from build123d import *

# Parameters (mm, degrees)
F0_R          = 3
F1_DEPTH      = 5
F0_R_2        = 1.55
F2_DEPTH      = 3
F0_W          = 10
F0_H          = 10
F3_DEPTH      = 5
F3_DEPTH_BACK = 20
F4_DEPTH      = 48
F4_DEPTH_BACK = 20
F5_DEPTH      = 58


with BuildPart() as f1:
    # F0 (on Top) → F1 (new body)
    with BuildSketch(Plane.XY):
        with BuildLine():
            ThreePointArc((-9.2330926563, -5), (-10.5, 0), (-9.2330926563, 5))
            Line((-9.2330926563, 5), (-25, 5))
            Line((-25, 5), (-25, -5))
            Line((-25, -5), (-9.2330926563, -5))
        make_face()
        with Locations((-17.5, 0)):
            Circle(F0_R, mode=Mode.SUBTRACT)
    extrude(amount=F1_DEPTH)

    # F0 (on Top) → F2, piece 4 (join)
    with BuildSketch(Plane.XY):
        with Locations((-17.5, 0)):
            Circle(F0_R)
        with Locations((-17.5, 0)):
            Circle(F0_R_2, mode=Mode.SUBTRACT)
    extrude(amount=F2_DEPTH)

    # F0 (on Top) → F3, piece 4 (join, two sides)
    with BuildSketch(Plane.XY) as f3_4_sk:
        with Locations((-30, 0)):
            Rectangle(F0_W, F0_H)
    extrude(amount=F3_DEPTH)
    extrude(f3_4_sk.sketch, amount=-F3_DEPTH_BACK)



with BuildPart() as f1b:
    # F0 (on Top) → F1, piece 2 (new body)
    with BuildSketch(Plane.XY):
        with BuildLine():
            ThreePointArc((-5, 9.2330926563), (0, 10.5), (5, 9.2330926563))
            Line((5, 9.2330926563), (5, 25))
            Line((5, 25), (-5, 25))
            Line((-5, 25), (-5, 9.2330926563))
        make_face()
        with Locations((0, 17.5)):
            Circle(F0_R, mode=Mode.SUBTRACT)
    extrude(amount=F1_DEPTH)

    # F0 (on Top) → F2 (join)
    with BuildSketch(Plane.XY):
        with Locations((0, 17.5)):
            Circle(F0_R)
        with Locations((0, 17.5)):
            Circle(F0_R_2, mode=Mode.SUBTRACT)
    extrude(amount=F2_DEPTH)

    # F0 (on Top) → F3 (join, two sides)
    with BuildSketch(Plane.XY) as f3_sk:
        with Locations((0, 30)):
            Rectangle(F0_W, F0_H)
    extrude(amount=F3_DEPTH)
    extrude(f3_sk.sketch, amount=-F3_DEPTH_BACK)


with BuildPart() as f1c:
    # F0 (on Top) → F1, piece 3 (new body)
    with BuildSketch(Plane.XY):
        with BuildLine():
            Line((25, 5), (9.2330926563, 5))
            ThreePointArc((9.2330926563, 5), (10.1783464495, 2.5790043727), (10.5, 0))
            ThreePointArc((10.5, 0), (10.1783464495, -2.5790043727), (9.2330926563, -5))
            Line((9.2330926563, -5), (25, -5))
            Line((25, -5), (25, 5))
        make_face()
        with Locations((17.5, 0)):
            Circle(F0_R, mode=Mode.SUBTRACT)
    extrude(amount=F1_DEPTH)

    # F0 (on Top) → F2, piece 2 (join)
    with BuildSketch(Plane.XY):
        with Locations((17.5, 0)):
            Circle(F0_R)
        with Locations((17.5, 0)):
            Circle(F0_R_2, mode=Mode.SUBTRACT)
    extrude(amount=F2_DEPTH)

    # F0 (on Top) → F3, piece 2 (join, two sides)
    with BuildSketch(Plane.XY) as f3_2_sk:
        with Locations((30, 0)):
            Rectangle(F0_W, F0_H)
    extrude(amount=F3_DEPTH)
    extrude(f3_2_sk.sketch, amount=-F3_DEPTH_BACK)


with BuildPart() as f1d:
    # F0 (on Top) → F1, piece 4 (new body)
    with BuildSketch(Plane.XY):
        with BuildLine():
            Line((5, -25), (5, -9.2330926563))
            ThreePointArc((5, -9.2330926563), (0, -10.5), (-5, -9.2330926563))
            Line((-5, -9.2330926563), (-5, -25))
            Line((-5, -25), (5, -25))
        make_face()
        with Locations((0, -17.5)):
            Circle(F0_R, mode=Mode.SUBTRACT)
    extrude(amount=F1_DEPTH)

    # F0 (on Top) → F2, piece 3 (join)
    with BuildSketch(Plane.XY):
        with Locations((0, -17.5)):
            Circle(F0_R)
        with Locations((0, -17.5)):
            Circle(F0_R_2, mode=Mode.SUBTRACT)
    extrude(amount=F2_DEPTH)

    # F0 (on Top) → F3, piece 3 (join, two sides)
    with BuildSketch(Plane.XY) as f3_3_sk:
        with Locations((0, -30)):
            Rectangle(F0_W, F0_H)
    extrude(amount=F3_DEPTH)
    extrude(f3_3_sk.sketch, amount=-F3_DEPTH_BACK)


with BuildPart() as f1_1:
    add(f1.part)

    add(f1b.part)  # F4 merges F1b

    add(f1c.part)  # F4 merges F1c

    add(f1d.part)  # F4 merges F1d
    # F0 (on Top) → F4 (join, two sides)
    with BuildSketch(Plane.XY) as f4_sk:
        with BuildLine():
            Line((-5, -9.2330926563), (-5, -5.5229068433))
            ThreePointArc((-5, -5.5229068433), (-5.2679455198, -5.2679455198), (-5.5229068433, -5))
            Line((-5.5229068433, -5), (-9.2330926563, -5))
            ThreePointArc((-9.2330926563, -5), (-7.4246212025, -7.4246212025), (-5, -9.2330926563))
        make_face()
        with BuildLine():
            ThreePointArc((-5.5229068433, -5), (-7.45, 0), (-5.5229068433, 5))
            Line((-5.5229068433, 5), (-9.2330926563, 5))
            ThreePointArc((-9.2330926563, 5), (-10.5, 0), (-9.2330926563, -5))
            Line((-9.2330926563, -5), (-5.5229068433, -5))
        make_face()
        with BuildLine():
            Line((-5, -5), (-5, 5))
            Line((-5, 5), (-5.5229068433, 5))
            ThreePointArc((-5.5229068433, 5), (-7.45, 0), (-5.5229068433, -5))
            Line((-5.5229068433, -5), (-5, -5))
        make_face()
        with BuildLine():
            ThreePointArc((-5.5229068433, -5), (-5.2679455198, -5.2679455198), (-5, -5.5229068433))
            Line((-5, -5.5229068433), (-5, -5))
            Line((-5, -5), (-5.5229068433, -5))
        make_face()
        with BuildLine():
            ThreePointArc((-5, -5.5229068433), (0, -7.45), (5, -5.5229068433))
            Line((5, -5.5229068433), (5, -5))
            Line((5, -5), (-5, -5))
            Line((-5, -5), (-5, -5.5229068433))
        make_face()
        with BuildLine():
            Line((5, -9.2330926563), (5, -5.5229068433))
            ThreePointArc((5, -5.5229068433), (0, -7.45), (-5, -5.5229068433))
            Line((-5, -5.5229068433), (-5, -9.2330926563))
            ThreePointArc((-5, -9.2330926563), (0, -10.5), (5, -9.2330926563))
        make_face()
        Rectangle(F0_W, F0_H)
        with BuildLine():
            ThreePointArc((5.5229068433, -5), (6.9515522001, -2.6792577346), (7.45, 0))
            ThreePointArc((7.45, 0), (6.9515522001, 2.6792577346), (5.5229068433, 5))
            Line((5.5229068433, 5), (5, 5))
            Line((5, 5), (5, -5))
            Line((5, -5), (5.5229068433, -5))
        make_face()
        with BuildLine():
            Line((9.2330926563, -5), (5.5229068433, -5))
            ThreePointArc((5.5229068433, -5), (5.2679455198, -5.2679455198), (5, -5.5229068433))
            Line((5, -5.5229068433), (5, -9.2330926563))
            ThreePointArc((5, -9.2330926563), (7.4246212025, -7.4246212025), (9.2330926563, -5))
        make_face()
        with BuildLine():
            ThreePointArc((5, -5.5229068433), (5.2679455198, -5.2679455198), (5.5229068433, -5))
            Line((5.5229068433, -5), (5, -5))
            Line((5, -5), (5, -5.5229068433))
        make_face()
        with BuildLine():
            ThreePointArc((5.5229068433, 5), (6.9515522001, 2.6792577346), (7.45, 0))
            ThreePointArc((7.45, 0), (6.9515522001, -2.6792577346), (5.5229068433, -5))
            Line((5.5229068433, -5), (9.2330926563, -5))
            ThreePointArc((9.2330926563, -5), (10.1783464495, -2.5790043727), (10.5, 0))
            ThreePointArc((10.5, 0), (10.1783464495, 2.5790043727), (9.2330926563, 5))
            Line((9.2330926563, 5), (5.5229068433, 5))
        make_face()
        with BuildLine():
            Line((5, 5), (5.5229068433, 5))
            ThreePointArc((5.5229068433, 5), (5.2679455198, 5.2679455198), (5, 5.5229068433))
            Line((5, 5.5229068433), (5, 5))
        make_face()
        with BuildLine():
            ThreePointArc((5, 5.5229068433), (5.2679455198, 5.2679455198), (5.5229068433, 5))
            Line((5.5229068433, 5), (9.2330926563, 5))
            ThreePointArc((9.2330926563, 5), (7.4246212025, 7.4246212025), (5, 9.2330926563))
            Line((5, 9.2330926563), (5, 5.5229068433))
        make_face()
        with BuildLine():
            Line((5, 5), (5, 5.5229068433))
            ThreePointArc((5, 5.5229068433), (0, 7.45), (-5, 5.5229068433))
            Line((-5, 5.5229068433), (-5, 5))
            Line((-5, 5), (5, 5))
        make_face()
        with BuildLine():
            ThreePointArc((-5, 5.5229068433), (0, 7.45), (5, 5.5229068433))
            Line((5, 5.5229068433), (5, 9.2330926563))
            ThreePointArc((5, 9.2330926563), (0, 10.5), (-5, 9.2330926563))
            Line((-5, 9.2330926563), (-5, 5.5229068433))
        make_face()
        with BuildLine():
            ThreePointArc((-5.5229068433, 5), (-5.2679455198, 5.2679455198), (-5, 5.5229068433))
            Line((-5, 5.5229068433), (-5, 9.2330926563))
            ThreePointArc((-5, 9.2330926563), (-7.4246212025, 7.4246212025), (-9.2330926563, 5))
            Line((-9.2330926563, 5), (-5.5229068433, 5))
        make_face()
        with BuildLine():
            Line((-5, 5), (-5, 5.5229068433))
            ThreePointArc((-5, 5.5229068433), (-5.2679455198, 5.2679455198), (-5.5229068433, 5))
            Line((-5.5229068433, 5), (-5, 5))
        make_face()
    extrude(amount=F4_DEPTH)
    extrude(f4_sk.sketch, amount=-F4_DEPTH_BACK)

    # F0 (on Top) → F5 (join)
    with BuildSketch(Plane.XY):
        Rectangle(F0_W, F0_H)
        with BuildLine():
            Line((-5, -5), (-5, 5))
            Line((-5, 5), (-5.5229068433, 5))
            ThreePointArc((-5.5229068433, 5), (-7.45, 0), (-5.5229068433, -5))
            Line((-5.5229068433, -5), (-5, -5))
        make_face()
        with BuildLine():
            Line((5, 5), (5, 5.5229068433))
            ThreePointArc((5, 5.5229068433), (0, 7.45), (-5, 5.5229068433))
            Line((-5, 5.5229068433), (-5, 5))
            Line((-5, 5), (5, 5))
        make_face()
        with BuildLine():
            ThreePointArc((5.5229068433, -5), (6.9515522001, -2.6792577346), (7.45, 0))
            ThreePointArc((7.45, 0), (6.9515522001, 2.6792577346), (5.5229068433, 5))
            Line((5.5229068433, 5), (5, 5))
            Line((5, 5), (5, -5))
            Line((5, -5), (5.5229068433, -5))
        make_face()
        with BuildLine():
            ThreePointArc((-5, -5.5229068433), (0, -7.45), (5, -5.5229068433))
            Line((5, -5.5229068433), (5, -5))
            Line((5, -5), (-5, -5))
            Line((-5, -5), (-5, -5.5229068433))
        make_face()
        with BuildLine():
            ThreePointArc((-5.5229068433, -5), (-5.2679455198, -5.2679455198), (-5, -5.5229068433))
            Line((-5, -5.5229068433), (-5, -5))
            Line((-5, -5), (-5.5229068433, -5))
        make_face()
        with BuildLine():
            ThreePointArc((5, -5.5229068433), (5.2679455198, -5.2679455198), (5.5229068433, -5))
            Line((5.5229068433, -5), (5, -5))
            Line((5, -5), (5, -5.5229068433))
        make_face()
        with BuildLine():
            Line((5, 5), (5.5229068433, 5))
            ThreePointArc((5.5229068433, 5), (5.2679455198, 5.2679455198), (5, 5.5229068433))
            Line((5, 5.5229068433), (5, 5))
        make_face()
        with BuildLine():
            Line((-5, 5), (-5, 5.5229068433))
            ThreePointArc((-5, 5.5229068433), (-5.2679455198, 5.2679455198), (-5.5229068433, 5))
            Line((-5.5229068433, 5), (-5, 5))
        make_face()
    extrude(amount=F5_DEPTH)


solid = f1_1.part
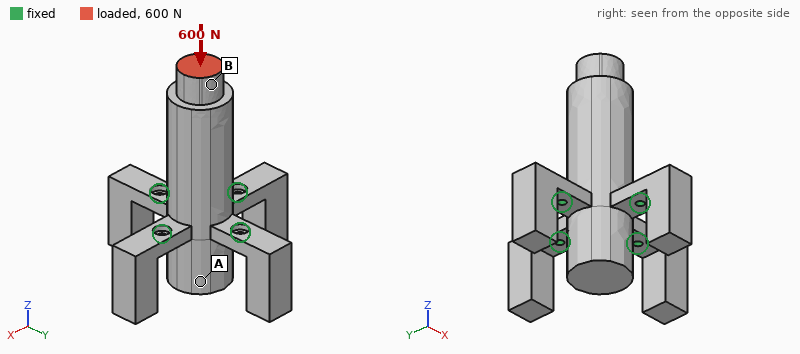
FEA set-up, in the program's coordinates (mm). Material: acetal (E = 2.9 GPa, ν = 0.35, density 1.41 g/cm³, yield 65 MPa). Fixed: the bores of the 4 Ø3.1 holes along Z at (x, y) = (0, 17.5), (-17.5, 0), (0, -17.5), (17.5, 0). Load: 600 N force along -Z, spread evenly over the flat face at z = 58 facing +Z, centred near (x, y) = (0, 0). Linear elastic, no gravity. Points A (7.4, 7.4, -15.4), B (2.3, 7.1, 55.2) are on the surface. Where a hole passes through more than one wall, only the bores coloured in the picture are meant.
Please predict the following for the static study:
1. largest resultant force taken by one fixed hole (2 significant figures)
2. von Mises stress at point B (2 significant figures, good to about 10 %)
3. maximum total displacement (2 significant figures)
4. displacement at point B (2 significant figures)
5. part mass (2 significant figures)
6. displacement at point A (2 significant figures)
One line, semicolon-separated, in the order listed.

170 N; 3.4 MPa; 0.10 mm; 0.098 mm; 54 g; 0.062 mm
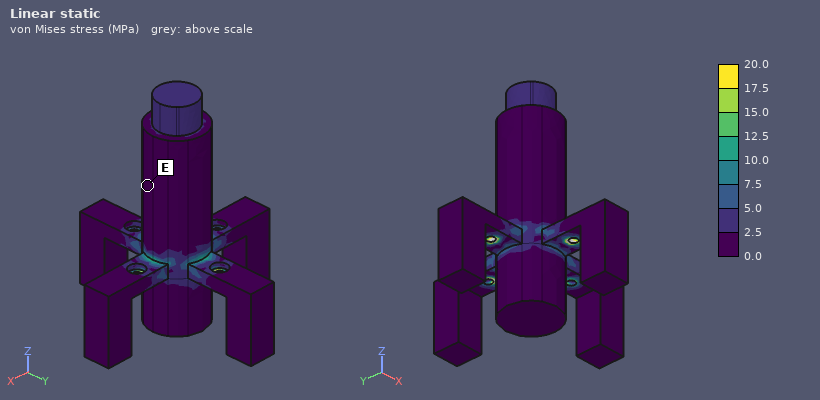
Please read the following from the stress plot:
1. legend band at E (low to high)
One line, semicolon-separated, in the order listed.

0.0 to 2.5 MPa
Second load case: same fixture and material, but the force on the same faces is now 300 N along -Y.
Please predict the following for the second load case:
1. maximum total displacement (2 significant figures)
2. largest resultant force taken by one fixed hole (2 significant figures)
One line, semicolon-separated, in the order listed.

1.5 mm; 570 N
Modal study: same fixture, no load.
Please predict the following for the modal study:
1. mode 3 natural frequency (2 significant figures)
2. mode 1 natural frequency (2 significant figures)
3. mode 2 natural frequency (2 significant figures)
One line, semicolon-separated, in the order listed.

840 Hz; 810 Hz; 820 Hz
